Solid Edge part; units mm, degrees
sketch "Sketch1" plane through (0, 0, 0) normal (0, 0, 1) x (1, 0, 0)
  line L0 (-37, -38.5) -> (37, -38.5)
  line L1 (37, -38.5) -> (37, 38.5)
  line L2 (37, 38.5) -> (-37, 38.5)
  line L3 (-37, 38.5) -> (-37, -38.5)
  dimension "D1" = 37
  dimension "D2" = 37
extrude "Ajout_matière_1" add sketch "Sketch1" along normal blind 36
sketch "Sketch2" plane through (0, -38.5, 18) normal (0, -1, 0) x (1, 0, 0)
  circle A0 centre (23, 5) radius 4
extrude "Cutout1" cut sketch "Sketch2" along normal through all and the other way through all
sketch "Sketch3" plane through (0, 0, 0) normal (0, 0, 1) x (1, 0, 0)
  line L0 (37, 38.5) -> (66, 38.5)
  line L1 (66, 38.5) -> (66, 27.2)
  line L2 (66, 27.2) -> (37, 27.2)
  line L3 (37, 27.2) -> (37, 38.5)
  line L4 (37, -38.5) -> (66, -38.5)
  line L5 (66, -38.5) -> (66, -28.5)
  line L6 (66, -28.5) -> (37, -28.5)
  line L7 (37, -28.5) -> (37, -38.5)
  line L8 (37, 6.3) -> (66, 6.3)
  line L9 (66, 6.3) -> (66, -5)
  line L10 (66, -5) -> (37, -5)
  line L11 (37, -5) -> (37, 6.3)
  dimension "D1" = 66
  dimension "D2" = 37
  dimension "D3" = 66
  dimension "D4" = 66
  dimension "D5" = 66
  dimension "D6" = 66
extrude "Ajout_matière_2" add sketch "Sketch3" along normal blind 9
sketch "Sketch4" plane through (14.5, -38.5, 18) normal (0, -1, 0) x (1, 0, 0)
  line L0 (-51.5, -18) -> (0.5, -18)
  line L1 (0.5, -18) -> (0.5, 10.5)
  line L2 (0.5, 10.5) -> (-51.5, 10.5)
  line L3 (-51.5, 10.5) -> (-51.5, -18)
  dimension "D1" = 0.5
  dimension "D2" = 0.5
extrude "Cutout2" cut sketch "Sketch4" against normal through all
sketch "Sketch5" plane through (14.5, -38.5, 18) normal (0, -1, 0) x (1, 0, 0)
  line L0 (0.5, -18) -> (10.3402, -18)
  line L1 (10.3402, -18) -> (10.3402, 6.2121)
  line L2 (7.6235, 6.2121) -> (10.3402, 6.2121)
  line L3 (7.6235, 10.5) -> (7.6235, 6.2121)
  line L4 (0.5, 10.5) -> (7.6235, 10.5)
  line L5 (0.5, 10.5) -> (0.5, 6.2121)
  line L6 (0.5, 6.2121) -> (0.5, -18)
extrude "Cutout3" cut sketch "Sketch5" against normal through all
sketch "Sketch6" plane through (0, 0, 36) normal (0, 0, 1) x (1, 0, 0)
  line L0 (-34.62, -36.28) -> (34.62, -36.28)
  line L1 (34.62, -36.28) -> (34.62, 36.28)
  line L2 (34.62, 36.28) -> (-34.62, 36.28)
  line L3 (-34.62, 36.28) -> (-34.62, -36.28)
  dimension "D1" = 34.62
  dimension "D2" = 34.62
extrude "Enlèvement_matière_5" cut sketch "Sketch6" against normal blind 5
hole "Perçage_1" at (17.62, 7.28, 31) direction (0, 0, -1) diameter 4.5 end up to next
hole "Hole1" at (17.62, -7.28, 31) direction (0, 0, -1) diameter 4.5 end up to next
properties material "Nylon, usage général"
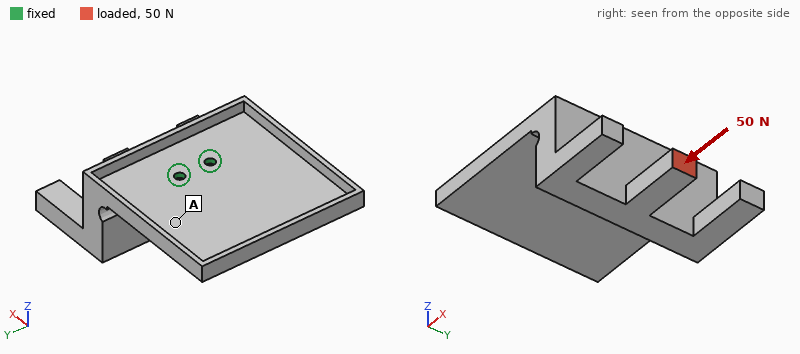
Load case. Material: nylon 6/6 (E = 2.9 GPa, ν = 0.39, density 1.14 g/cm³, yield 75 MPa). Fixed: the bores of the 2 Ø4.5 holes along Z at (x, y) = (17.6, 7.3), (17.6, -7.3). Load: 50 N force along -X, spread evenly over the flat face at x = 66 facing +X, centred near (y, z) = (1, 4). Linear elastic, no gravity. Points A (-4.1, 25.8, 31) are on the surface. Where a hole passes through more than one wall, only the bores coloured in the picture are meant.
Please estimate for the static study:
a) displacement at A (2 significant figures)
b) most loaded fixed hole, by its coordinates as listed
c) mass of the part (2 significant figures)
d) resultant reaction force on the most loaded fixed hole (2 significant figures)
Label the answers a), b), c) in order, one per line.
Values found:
a) 0.46 mm
b) (17.6, 7.3)
c) 60 g
d) 27 N
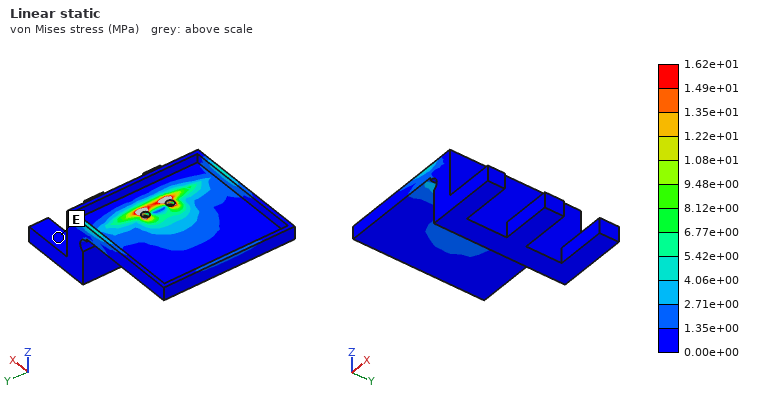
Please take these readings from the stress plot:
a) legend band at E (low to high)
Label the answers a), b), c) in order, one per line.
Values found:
a) 0.00e+00 to 1.35e+00 MPa
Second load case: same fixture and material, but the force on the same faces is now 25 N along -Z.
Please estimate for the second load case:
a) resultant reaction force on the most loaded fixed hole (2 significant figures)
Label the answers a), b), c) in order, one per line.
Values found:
a) 15 N
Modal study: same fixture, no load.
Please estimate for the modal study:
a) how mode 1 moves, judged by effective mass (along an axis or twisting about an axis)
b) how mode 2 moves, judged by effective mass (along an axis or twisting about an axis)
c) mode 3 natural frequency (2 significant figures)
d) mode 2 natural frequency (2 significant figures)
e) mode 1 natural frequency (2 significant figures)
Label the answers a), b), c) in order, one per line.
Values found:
a) along X
b) along Z
c) 370 Hz
d) 320 Hz
e) 160 Hz
